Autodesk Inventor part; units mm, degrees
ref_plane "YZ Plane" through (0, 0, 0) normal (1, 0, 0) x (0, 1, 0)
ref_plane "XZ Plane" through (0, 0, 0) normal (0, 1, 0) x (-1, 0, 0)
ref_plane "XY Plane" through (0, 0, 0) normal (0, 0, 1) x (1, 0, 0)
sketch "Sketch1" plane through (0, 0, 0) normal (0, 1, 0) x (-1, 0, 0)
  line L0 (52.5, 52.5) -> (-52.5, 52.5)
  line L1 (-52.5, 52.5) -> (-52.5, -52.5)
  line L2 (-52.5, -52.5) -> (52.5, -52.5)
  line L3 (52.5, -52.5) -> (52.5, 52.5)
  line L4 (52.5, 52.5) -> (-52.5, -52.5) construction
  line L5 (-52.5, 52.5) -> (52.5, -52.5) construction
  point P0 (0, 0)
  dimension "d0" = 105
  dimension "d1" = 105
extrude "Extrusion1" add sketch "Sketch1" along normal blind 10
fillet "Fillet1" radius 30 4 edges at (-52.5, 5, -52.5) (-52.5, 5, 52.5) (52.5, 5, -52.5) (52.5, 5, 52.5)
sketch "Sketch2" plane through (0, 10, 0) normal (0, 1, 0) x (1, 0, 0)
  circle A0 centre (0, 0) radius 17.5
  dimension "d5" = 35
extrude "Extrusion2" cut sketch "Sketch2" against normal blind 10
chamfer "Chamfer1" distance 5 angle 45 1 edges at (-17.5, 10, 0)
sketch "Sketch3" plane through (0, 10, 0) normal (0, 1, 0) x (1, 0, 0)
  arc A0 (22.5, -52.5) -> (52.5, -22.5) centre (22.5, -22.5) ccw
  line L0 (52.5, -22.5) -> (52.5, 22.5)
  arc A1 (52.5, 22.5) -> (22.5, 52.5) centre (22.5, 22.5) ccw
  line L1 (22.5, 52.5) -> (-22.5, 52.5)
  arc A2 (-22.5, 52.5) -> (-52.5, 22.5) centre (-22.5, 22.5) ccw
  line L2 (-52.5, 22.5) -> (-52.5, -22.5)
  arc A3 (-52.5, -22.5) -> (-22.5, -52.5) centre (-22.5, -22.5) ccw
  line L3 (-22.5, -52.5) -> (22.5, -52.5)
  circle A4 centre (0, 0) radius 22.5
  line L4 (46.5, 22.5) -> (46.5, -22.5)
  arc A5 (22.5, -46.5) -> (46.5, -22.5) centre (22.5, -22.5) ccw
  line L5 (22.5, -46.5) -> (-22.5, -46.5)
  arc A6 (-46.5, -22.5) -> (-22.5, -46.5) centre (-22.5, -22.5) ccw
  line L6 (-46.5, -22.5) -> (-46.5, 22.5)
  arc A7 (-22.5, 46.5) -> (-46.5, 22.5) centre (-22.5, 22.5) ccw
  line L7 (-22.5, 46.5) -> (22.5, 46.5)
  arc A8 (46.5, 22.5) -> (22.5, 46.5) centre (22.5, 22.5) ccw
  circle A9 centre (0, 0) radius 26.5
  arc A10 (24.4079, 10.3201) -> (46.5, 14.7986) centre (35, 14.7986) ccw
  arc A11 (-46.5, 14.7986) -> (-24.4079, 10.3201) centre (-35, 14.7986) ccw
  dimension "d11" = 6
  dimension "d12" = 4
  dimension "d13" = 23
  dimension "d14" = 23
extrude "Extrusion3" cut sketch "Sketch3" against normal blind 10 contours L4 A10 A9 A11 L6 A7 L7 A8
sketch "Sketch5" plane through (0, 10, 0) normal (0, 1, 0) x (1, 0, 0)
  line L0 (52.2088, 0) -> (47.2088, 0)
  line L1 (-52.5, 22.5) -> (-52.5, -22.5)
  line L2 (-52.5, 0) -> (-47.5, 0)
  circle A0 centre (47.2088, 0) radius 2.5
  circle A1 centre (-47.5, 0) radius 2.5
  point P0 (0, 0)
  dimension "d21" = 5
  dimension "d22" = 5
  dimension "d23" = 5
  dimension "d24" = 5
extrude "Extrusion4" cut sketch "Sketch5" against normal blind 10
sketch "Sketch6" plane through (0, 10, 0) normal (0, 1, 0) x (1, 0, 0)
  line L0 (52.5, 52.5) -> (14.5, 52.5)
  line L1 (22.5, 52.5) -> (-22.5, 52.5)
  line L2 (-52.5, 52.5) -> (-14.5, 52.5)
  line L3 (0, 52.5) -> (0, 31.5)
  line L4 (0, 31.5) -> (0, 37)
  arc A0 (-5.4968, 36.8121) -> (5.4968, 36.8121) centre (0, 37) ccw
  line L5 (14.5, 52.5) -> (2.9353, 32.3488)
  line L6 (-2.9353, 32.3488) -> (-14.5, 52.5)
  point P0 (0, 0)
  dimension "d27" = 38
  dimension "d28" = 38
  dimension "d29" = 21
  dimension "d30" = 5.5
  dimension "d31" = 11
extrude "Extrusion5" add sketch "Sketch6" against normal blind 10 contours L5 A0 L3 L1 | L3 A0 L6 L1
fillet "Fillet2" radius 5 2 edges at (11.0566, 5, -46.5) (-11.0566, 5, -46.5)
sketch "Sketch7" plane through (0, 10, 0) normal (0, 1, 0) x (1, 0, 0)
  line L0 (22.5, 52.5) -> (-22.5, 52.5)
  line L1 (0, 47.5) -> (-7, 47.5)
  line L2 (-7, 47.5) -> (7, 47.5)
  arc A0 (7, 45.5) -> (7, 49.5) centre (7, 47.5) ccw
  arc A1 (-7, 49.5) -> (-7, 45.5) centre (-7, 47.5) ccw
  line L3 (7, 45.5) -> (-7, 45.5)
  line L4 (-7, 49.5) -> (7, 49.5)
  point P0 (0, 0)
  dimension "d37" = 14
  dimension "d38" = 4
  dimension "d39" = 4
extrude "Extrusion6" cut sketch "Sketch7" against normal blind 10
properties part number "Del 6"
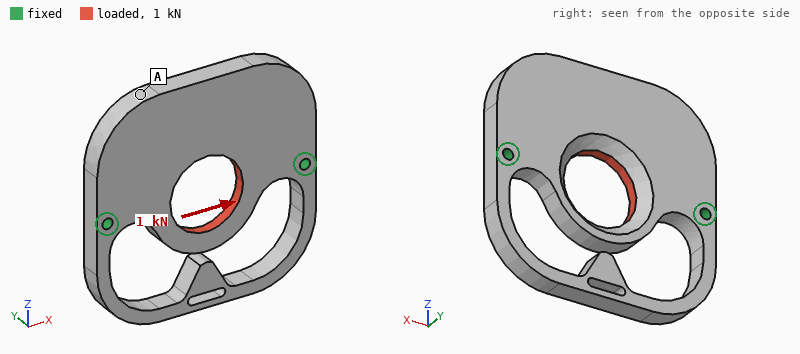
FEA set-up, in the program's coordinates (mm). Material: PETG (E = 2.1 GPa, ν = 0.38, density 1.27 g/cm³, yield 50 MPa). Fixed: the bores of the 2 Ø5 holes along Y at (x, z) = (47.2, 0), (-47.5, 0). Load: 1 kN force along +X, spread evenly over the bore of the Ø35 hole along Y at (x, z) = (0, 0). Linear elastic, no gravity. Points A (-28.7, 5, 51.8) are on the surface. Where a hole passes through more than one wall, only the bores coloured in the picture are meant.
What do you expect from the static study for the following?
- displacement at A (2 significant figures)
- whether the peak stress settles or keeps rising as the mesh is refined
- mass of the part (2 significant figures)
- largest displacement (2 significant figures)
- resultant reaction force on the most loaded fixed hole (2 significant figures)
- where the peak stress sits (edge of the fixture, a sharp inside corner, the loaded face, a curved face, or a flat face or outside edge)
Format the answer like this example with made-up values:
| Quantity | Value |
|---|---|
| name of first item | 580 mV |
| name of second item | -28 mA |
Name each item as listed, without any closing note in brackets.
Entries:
| Quantity | Value |
|---|---|
| displacement at A | 0.035 mm |
| whether the peak stress settles or keeps rising as the mesh is refined | keeps rising |
| mass of the part | 82 g |
| largest displacement | 0.17 mm |
| resultant reaction force on the most loaded fixed hole | 500 N |
| where the peak stress sits | edge of the fixture |
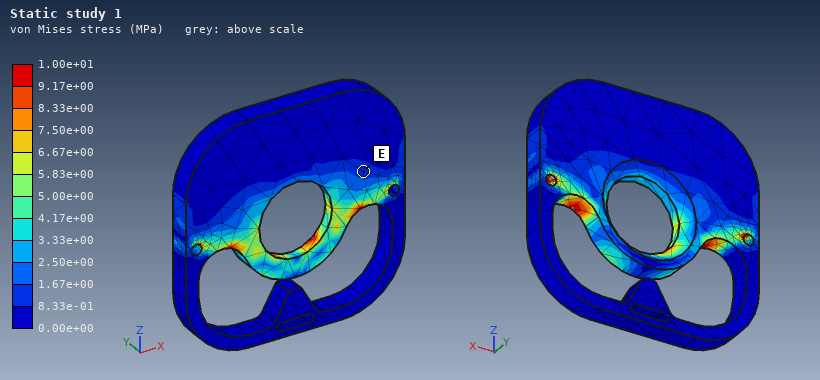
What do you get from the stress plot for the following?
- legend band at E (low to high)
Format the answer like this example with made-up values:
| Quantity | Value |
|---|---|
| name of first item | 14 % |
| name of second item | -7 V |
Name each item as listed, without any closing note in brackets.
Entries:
| Quantity | Value |
|---|---|
| legend band at E | 8.33e-01 to 1.67e+00 MPa |
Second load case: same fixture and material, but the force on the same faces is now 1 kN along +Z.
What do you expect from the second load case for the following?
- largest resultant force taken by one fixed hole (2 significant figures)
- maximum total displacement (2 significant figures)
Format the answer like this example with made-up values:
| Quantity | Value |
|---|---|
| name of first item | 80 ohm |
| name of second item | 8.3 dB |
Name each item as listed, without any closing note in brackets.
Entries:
| Quantity | Value |
|---|---|
| largest resultant force taken by one fixed hole | 540 N |
| maximum total displacement | 0.42 mm |
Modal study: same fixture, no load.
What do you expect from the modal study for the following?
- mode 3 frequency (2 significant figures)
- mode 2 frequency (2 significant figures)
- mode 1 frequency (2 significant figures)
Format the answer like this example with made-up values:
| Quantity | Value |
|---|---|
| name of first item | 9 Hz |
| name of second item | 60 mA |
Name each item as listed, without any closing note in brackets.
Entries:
| Quantity | Value |
|---|---|
| mode 3 frequency | 460 Hz |
| mode 2 frequency | 460 Hz |
| mode 1 frequency | 360 Hz |
